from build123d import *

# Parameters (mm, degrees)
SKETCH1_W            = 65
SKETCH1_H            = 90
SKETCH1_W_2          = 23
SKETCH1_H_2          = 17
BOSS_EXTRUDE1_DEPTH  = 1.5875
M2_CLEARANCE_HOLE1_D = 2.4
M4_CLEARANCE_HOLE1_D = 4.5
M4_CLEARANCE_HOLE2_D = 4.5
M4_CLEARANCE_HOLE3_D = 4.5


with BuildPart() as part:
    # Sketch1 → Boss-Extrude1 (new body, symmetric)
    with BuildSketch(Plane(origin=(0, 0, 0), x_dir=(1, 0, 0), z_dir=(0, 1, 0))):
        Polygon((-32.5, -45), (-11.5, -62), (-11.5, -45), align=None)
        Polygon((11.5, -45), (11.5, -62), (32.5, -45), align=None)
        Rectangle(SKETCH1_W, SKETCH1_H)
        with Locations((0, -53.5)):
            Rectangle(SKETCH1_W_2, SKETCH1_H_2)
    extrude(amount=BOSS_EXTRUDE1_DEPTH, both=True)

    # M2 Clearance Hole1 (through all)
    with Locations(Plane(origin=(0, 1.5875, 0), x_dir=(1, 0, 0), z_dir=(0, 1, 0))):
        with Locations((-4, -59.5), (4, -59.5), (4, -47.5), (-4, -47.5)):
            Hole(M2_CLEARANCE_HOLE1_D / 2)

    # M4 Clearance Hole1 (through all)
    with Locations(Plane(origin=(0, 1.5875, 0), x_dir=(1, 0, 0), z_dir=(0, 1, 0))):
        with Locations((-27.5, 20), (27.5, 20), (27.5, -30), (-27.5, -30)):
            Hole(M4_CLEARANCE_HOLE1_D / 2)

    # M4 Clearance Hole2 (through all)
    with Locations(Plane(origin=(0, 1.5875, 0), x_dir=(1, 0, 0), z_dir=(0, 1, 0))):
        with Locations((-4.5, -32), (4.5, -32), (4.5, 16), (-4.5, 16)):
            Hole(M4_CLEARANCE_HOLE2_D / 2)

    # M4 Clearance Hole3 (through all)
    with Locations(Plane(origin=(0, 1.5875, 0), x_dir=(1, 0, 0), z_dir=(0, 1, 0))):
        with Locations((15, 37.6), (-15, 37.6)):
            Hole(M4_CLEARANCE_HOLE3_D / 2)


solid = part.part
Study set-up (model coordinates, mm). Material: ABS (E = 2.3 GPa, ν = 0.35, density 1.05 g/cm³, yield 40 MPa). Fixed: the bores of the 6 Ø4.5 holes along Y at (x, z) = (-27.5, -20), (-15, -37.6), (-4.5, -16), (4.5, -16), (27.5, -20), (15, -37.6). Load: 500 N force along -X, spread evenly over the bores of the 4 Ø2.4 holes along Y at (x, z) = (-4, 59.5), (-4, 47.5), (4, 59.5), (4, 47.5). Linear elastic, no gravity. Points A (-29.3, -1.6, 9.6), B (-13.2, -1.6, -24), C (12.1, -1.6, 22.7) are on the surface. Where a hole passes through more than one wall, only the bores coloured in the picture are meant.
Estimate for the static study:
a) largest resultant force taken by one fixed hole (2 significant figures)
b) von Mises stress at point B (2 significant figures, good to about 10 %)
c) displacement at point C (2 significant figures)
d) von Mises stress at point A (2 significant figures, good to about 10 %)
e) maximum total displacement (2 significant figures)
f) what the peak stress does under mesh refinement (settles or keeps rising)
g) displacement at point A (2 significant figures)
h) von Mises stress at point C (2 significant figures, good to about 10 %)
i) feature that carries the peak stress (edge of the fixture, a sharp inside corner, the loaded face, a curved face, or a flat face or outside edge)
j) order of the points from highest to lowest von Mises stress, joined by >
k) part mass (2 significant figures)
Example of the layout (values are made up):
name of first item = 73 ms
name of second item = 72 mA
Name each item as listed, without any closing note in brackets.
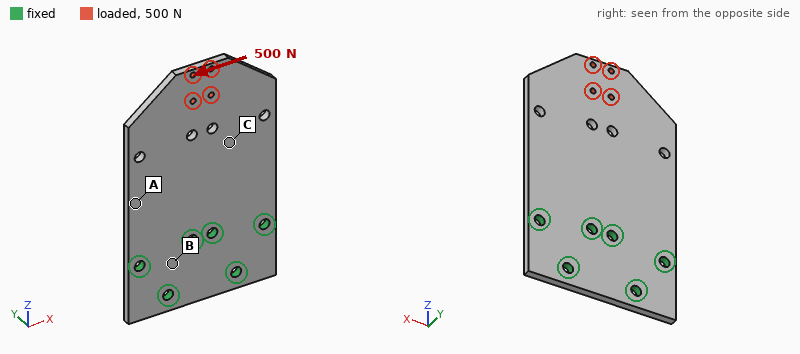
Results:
largest resultant force taken by one fixed hole = 570 N
von Mises stress at point B = 2.4 MPa
displacement at point C = 0.30 mm
von Mises stress at point A = 9.1 MPa
maximum total displacement = 0.74 mm
what the peak stress does under mesh refinement = keeps rising
displacement at point A = 0.24 mm
von Mises stress at point C = 5.5 MPa
feature that carries the peak stress = edge of the fixture
order of the points from highest to lowest von Mises stress, joined by > = A > C > B
part mass = 21 g
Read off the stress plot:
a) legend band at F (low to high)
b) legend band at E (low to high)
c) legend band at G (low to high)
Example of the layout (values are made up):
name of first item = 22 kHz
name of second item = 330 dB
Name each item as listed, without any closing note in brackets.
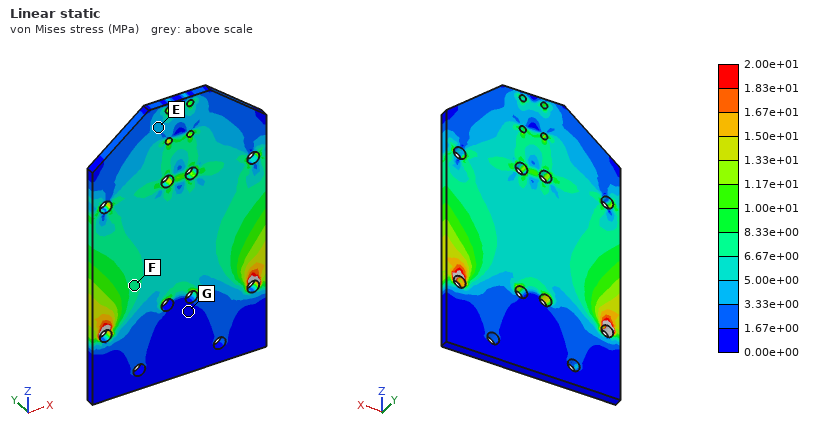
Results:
legend band at F = 6.67e+00 to 8.33e+00 MPa
legend band at E = 3.33e+00 to 5.00e+00 MPa
legend band at G = 0.00e+00 to 1.67e+00 MPa
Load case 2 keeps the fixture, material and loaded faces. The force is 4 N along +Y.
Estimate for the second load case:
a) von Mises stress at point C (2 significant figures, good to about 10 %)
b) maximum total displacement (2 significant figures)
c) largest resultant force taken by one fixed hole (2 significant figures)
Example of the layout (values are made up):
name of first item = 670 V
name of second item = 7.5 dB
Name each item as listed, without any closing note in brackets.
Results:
von Mises stress at point C = 1.1 MPa
maximum total displacement = 1.3 mm
largest resultant force taken by one fixed hole = 4.1 N
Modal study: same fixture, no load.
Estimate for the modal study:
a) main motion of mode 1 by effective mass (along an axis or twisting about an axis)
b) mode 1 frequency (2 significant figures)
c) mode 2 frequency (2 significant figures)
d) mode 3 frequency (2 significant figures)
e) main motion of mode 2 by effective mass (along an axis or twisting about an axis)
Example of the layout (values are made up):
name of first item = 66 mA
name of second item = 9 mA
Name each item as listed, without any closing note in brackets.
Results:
main motion of mode 1 by effective mass = along Y
mode 1 frequency = 150 Hz
mode 2 frequency = 400 Hz
mode 3 frequency = 800 Hz
main motion of mode 2 by effective mass = twisting about Z
